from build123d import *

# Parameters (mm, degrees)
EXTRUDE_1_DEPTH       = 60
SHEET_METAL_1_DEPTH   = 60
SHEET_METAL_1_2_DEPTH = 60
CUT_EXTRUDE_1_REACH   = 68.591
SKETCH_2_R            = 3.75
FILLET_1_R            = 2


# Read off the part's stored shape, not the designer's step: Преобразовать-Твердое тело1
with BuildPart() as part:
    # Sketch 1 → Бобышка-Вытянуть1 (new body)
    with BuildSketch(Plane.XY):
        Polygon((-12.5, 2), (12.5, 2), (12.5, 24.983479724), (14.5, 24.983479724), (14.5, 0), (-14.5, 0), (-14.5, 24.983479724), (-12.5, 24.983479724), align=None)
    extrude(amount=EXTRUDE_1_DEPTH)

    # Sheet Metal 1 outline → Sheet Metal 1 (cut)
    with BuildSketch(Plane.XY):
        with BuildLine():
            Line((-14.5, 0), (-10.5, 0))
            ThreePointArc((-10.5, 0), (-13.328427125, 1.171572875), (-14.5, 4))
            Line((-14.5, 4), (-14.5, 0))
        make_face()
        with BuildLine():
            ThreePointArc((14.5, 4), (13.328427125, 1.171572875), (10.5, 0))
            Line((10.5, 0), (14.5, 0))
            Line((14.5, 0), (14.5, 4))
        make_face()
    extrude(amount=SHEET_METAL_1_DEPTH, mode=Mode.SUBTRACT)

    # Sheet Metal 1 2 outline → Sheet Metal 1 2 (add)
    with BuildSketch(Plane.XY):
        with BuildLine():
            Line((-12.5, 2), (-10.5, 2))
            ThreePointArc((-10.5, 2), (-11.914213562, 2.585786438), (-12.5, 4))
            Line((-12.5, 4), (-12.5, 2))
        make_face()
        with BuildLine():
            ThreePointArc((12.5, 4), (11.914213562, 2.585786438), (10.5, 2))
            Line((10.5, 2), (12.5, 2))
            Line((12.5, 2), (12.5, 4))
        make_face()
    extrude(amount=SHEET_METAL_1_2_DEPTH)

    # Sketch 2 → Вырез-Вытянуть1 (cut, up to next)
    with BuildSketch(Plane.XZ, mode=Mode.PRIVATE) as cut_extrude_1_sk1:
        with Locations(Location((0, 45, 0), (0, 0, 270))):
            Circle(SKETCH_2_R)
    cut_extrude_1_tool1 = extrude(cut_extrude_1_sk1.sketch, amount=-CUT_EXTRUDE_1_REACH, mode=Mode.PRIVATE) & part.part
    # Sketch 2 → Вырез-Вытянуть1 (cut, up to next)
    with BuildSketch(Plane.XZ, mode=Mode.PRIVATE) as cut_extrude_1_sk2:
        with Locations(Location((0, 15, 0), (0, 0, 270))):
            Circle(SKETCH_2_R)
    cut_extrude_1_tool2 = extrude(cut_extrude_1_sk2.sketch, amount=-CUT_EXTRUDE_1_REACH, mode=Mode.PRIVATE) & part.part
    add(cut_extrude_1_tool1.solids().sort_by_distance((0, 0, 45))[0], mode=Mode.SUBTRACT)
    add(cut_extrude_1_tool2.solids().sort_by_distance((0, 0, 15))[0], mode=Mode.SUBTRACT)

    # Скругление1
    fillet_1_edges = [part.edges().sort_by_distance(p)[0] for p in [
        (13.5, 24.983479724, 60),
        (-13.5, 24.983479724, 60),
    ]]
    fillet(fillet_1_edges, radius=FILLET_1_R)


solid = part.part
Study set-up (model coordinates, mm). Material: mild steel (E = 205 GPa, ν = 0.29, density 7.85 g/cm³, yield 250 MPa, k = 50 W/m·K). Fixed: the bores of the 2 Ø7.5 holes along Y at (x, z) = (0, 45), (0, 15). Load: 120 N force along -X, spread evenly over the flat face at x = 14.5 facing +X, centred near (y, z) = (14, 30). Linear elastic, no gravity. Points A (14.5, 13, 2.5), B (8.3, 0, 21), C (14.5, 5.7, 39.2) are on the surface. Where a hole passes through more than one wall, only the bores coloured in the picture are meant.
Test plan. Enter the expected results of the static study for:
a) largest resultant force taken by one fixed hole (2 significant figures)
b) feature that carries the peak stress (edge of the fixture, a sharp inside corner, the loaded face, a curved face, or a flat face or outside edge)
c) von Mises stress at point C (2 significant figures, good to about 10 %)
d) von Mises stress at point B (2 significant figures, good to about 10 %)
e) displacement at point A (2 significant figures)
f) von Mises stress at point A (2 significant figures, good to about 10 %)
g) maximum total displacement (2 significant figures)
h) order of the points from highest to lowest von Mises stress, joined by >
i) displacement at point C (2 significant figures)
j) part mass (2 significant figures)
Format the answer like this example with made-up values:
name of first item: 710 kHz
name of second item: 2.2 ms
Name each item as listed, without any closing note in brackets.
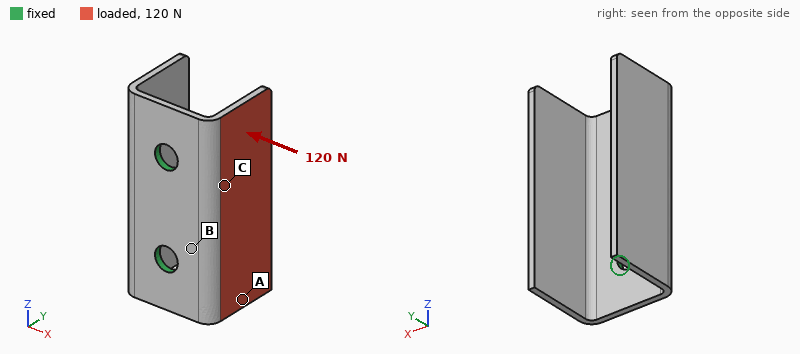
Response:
largest resultant force taken by one fixed hole: 60 N
feature that carries the peak stress: a flat face or outside edge
von Mises stress at point C: 24 MPa
von Mises stress at point B: 37 MPa
displacement at point A: 36 µm
von Mises stress at point A: 10 MPa
maximum total displacement: 75 µm
order of the points from highest to lowest von Mises stress, joined by >: B > C > A
displacement at point C: 19 µm
part mass: 67 g
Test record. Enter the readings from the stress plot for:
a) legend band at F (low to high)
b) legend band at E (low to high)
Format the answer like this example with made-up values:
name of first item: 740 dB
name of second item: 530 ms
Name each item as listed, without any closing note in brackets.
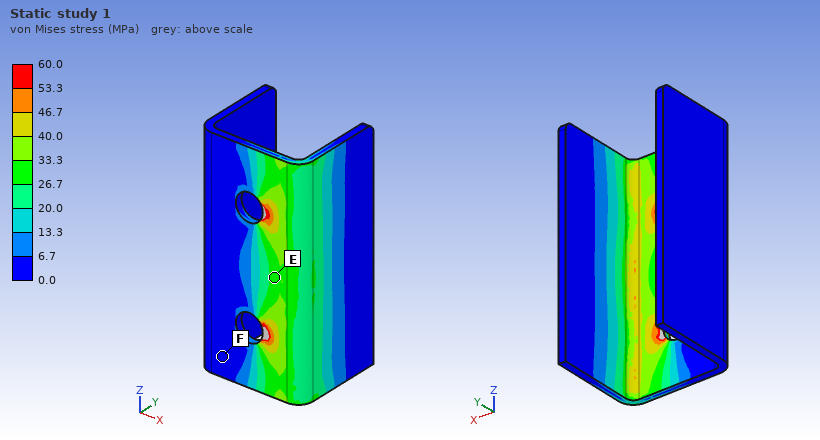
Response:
legend band at F: 0.0 to 6.7 MPa
legend band at E: 26.7 to 33.3 MPa
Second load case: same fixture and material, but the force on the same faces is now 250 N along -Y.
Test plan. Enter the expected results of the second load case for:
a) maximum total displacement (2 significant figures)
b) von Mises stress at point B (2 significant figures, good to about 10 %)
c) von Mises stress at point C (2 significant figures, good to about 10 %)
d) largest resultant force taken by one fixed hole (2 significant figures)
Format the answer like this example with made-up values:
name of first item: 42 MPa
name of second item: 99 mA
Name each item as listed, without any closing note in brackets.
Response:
maximum total displacement: 65 µm
von Mises stress at point B: 39 MPa
von Mises stress at point C: 6.8 MPa
largest resultant force taken by one fixed hole: 130 N
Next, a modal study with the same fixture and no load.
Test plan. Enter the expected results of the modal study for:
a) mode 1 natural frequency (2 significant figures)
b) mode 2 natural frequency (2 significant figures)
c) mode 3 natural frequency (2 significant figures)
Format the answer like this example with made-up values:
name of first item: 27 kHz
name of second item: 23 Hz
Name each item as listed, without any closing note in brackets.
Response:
mode 1 natural frequency: 1700 Hz
mode 2 natural frequency: 1700 Hz
mode 3 natural frequency: 2600 Hz
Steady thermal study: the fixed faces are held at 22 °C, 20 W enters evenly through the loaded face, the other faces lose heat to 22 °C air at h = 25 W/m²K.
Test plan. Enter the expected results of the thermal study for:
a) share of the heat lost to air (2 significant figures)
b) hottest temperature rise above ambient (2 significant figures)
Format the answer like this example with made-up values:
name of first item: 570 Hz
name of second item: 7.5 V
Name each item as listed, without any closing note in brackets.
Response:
share of the heat lost to air: 20 %
hottest temperature rise above ambient: 74 K
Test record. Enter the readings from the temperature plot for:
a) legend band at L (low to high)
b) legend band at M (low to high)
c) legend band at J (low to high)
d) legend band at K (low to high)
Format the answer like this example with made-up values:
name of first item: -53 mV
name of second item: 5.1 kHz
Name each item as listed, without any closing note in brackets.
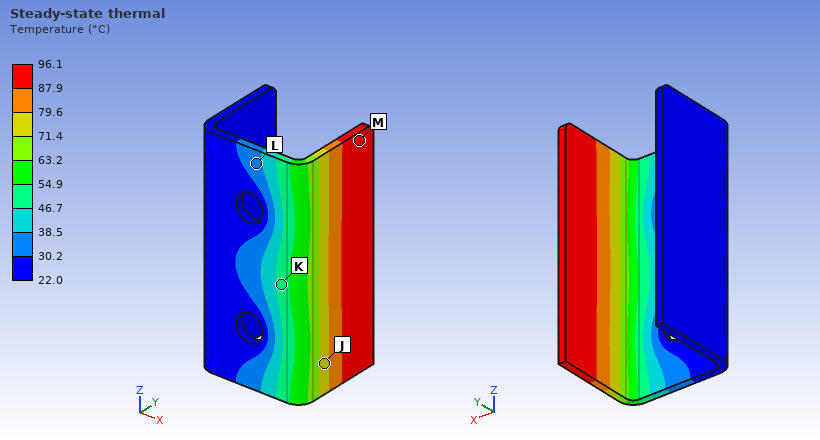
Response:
legend band at L: 30.2 to 38.5 °C
legend band at M: 87.9 to 96.1 °C
legend band at J: 71.4 to 79.6 °C
legend band at K: 46.7 to 54.9 °C
